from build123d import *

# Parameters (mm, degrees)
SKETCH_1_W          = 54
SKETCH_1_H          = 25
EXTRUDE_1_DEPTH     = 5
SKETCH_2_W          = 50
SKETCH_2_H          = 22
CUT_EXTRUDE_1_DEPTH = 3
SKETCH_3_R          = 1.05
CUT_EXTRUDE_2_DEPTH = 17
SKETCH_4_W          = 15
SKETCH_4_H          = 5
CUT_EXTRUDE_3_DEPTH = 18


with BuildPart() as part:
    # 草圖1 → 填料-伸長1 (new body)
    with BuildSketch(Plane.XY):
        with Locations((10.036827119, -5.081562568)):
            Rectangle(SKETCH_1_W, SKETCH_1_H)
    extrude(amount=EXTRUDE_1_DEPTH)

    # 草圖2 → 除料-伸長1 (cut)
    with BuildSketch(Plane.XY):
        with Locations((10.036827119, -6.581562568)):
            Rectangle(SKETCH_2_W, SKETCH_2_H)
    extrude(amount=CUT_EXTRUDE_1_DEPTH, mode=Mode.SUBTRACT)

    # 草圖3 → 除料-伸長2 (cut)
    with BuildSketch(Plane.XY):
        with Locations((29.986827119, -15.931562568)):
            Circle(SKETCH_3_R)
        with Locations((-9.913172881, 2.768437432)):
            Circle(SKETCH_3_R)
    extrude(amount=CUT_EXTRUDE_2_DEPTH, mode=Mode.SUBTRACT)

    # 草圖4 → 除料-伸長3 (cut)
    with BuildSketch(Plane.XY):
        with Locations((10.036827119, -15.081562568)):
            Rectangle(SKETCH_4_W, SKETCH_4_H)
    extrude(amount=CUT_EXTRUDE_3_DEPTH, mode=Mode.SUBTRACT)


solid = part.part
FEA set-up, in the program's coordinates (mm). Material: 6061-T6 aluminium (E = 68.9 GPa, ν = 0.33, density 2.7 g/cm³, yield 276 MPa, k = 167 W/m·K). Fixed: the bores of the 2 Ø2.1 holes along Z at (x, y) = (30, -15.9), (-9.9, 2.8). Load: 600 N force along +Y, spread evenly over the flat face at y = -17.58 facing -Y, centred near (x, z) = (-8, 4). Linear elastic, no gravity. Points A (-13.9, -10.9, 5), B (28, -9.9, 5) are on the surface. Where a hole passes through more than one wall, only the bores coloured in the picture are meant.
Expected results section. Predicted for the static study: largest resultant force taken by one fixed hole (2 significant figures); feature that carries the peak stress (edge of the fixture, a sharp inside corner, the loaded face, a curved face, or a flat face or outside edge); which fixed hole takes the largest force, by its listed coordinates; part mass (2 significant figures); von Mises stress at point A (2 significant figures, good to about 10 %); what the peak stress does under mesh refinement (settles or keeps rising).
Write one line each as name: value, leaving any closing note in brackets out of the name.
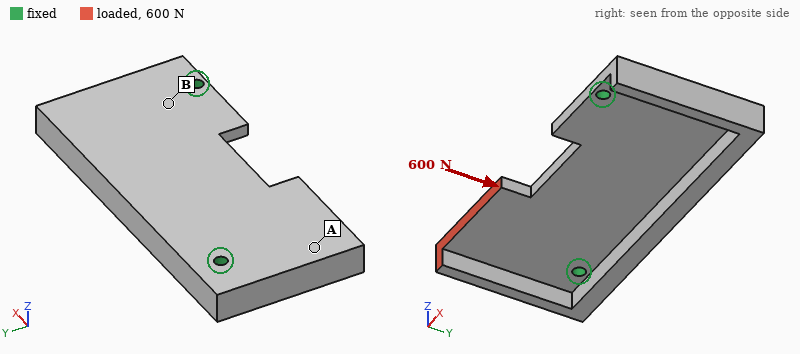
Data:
largest resultant force taken by one fixed hole: 560 N
feature that carries the peak stress: edge of the fixture
which fixed hole takes the largest force, by its listed coordinates: (-9.9, 2.8)
part mass: 8.9 g
von Mises stress at point A: 14 MPa
what the peak stress does under mesh refinement: keeps rising
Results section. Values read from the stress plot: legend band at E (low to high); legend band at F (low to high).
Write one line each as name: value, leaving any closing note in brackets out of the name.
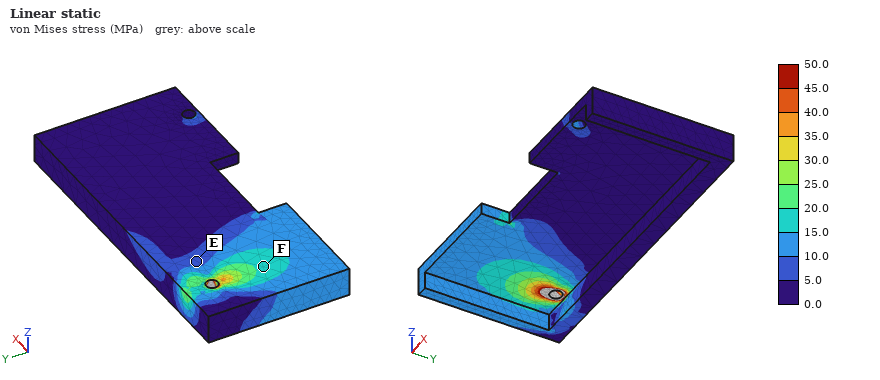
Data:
legend band at E: 5.0 to 10.0 MPa
legend band at F: 15.0 to 20.0 MPa
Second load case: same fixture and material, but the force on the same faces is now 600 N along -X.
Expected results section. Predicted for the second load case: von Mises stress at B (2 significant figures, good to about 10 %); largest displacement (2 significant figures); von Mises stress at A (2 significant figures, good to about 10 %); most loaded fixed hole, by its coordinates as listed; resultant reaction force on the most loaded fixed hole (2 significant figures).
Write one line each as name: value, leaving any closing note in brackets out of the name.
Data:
von Mises stress at B: 20 MPa
largest displacement: 65 µm
von Mises stress at A: 20 MPa
most loaded fixed hole, by its coordinates as listed: (-9.9, 2.8)
resultant reaction force on the most loaded fixed hole: 560 N
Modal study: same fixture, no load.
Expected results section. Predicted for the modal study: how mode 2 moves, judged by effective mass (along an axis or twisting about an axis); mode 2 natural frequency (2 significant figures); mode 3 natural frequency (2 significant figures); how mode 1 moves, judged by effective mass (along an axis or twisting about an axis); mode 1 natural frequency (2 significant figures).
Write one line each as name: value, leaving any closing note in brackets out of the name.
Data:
how mode 2 moves, judged by effective mass: along Z
mode 2 natural frequency: 4400 Hz
mode 3 natural frequency: 6600 Hz
how mode 1 moves, judged by effective mass: along Z
mode 1 natural frequency: 2900 Hz
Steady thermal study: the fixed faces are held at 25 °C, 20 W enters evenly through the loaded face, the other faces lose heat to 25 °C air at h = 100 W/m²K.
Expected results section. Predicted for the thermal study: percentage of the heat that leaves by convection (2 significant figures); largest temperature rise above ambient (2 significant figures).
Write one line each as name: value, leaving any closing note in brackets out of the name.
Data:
percentage of the heat that leaves by convection: 22 %
largest temperature rise above ambient: 51 K
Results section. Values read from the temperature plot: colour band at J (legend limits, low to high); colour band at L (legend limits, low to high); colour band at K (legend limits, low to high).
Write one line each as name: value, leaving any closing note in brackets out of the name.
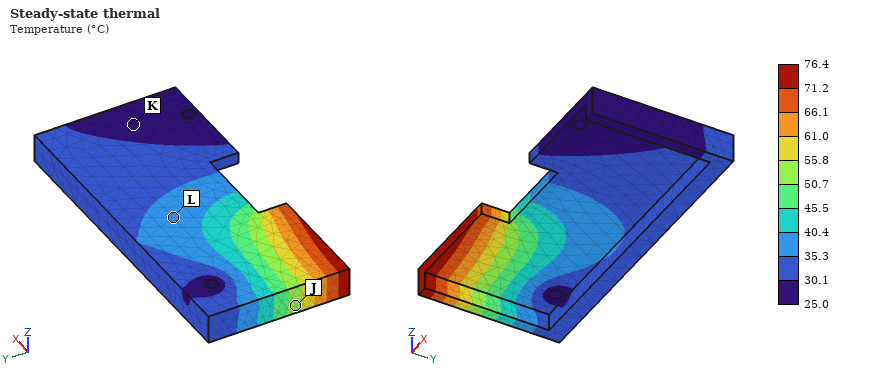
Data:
colour band at J: 50.7 to 55.8 °C
colour band at L: 35.3 to 40.4 °C
colour band at K: 25.0 to 30.1 °C
